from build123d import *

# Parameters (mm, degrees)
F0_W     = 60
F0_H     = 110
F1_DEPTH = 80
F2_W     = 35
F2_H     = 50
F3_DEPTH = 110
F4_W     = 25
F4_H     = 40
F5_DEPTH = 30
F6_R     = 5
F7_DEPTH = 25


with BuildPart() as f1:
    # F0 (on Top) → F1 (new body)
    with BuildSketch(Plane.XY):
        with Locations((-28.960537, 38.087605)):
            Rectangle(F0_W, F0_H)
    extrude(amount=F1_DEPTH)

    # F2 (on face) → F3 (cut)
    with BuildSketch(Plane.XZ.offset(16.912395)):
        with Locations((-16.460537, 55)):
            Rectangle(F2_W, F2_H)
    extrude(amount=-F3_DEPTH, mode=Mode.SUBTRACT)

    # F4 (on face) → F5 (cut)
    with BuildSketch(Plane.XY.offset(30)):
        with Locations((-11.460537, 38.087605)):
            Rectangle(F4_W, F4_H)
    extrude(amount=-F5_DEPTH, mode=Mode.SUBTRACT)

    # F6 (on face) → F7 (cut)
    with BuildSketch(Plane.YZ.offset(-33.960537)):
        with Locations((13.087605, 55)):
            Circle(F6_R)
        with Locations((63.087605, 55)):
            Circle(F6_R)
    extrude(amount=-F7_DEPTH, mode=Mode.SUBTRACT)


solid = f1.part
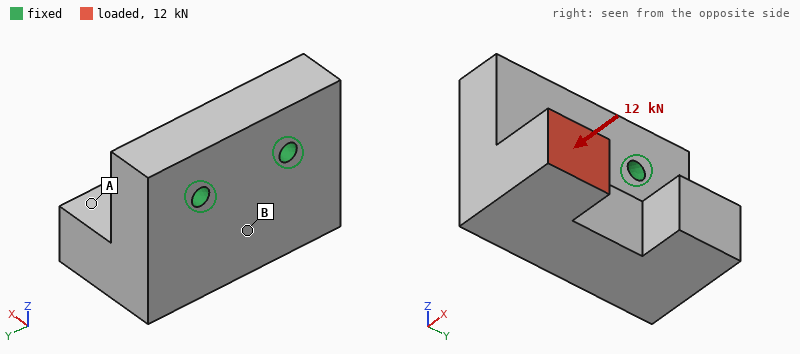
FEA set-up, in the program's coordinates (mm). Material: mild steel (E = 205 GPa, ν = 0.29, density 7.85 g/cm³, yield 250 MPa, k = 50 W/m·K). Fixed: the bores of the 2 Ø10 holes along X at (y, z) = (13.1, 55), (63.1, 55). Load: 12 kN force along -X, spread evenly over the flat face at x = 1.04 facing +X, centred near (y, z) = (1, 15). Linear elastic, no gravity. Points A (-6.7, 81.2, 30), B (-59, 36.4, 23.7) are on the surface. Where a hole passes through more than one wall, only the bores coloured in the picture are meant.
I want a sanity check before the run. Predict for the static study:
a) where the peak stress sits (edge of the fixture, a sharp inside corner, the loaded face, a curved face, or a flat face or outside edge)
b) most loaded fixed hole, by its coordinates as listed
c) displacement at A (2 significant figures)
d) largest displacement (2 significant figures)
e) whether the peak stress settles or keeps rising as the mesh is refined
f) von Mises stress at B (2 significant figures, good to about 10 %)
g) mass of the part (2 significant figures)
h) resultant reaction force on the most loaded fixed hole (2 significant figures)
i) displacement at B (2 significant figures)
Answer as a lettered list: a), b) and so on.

a) edge of the fixture
b) (13.1, 55)
c) 13 µm
d) 49 µm
e) keeps rising
f) 22 MPa
g) 2.4 kg
h) 12 kN
i) 11 µm
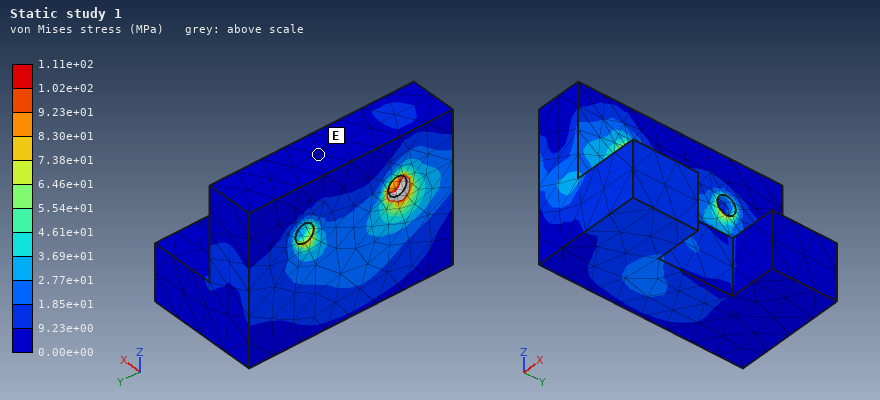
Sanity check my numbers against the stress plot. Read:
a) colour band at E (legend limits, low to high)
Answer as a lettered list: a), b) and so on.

a) 0.00e+00 to 9.23e+00 MPa
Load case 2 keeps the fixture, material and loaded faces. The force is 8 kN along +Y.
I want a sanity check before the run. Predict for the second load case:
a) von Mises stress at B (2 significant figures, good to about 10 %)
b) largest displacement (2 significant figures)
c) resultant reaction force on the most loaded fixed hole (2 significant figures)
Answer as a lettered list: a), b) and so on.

a) 13 MPa
b) 34 µm
c) 8.5 kN
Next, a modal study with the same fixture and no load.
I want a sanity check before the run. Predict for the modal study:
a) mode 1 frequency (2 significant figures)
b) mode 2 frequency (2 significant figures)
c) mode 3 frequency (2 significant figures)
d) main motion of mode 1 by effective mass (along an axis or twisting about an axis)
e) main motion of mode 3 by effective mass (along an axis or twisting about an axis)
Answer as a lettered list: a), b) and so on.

a) 3200 Hz
b) 4400 Hz
c) 6000 Hz
d) along X
e) along Y
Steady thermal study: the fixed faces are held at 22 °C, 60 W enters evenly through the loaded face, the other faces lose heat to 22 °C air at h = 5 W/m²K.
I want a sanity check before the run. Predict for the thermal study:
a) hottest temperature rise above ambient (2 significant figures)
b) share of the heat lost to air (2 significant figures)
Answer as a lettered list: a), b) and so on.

a) 69 K
b) 4.1 %
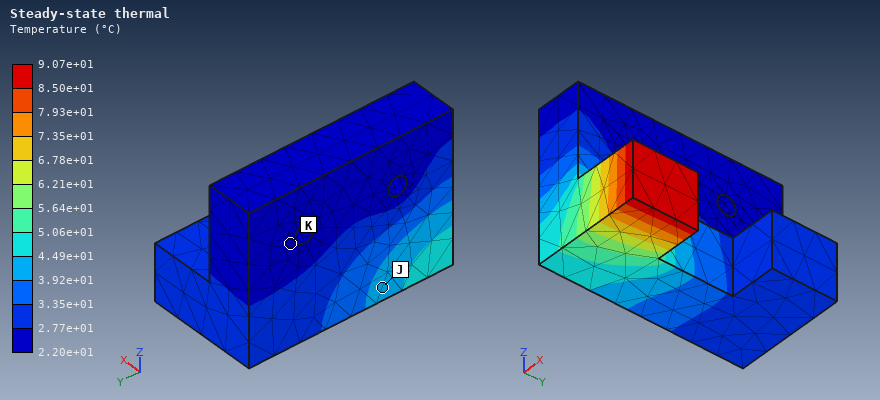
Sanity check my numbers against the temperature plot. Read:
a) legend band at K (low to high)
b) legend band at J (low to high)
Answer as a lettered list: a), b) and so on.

a) 2.20e+01 to 2.77e+01 °C
b) 3.92e+01 to 4.49e+01 °C
